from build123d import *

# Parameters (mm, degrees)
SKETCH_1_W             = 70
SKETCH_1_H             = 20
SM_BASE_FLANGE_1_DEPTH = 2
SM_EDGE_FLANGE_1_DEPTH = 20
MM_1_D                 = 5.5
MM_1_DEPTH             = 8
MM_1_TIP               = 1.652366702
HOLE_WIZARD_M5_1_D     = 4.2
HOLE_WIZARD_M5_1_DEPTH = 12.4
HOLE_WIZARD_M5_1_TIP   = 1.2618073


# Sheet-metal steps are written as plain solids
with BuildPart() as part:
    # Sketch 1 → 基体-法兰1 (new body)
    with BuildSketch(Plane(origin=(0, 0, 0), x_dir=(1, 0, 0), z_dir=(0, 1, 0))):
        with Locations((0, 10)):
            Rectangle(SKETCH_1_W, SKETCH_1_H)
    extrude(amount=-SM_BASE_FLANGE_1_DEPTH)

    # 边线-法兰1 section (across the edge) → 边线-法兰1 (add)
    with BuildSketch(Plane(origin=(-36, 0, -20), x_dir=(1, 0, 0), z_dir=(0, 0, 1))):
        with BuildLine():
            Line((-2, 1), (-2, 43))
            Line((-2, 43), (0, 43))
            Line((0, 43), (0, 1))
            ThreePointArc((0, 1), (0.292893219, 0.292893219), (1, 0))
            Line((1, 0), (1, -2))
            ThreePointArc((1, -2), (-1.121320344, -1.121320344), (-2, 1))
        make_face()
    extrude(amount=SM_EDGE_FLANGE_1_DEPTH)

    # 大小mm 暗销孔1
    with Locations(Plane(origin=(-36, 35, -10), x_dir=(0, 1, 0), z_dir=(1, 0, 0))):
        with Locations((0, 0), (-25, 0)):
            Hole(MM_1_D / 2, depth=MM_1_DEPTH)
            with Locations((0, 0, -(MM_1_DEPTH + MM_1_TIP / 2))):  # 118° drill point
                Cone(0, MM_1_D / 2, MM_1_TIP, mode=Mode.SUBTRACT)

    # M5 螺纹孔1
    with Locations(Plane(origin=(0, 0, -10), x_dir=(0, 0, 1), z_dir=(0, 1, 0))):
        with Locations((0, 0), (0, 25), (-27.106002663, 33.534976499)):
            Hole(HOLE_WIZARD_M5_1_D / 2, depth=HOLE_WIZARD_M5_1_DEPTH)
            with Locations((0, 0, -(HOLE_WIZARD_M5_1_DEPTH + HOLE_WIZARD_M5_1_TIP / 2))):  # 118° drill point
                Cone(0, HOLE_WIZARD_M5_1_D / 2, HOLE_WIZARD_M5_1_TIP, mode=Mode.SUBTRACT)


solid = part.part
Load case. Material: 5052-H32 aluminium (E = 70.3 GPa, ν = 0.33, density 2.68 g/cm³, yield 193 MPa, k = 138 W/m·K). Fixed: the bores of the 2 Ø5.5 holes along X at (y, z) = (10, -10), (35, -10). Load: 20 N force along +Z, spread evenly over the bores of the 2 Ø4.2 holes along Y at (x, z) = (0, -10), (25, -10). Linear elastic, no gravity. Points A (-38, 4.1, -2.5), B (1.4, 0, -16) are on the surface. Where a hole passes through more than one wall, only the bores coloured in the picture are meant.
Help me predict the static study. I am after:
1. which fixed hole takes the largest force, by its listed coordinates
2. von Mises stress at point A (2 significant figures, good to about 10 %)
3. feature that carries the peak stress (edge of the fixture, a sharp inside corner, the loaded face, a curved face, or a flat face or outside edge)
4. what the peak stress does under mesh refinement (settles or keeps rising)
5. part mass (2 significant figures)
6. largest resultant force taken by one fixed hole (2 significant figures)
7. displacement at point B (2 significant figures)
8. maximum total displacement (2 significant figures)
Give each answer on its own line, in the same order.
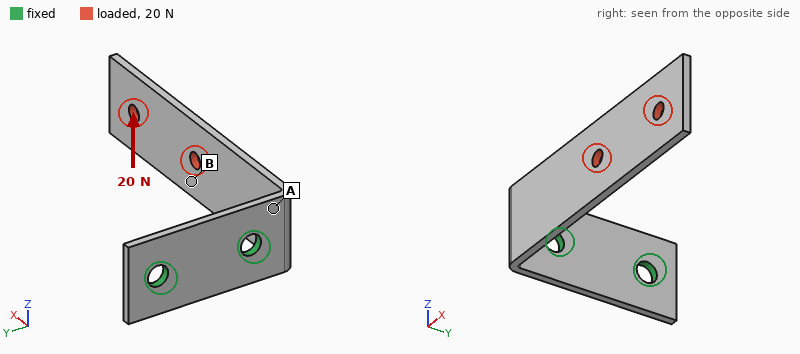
(10, -10)
27 MPa
edge of the fixture
keeps rising
12 g
25 N
0.19 mm
0.36 mm
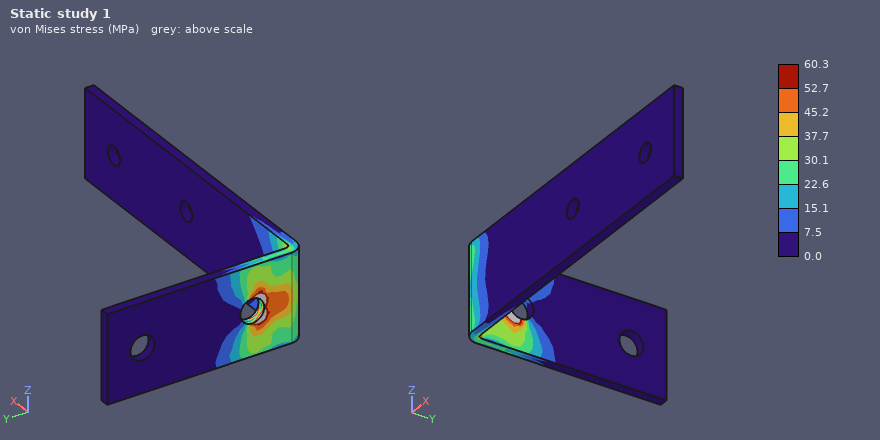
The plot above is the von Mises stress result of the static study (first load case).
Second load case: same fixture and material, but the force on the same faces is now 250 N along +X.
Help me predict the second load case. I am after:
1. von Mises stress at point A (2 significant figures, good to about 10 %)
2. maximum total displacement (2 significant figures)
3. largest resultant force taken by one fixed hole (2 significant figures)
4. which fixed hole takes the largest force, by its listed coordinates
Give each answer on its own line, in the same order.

73 MPa
0.86 mm
260 N
(10, -10)
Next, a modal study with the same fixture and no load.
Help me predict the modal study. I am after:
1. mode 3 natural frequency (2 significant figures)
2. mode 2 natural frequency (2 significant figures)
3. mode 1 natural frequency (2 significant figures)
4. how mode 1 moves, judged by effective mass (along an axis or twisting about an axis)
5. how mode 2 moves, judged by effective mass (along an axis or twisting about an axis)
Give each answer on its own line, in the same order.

1700 Hz
620 Hz
270 Hz
along Y
along Z
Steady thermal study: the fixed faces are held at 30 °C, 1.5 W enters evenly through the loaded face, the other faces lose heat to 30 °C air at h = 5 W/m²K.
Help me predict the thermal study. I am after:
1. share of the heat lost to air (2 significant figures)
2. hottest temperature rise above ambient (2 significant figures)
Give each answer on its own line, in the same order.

11 %
15 K
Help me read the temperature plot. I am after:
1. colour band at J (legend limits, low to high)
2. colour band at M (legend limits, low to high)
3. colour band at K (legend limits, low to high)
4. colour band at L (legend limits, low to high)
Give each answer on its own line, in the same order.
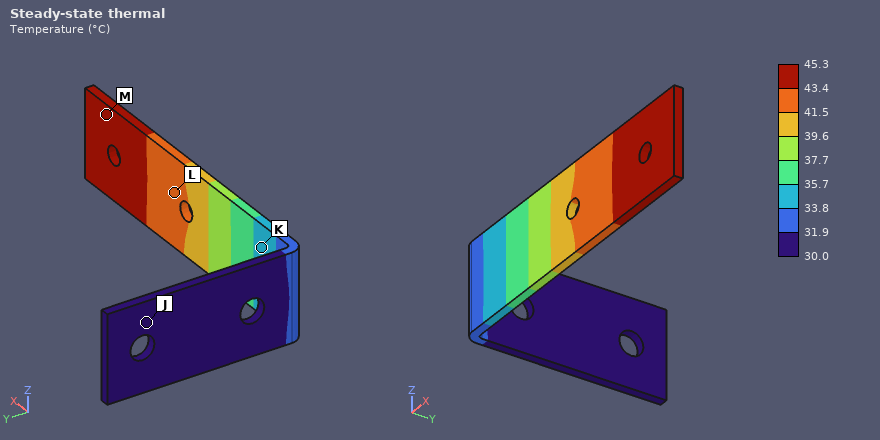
30.0 to 31.9 °C
43.4 to 45.3 °C
33.8 to 35.7 °C
41.5 to 43.4 °C
